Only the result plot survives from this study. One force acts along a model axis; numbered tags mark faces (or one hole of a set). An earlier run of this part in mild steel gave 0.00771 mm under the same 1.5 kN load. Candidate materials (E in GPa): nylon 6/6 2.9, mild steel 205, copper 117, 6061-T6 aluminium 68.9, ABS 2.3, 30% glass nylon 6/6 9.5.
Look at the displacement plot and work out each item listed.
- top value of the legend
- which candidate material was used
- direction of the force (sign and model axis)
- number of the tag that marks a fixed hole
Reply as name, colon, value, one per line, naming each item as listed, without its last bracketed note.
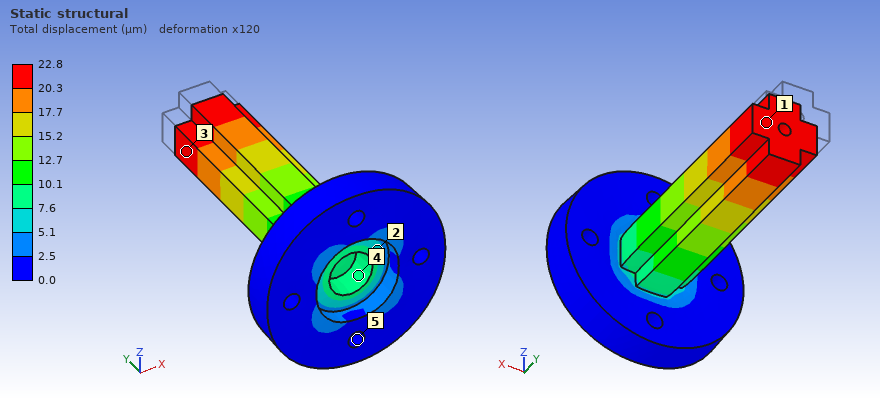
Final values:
top value of the legend: 22.8 µm
which candidate material was used: 6061-T6 aluminium
direction of the force: -Y
number of the tag that marks a fixed hole: 5
